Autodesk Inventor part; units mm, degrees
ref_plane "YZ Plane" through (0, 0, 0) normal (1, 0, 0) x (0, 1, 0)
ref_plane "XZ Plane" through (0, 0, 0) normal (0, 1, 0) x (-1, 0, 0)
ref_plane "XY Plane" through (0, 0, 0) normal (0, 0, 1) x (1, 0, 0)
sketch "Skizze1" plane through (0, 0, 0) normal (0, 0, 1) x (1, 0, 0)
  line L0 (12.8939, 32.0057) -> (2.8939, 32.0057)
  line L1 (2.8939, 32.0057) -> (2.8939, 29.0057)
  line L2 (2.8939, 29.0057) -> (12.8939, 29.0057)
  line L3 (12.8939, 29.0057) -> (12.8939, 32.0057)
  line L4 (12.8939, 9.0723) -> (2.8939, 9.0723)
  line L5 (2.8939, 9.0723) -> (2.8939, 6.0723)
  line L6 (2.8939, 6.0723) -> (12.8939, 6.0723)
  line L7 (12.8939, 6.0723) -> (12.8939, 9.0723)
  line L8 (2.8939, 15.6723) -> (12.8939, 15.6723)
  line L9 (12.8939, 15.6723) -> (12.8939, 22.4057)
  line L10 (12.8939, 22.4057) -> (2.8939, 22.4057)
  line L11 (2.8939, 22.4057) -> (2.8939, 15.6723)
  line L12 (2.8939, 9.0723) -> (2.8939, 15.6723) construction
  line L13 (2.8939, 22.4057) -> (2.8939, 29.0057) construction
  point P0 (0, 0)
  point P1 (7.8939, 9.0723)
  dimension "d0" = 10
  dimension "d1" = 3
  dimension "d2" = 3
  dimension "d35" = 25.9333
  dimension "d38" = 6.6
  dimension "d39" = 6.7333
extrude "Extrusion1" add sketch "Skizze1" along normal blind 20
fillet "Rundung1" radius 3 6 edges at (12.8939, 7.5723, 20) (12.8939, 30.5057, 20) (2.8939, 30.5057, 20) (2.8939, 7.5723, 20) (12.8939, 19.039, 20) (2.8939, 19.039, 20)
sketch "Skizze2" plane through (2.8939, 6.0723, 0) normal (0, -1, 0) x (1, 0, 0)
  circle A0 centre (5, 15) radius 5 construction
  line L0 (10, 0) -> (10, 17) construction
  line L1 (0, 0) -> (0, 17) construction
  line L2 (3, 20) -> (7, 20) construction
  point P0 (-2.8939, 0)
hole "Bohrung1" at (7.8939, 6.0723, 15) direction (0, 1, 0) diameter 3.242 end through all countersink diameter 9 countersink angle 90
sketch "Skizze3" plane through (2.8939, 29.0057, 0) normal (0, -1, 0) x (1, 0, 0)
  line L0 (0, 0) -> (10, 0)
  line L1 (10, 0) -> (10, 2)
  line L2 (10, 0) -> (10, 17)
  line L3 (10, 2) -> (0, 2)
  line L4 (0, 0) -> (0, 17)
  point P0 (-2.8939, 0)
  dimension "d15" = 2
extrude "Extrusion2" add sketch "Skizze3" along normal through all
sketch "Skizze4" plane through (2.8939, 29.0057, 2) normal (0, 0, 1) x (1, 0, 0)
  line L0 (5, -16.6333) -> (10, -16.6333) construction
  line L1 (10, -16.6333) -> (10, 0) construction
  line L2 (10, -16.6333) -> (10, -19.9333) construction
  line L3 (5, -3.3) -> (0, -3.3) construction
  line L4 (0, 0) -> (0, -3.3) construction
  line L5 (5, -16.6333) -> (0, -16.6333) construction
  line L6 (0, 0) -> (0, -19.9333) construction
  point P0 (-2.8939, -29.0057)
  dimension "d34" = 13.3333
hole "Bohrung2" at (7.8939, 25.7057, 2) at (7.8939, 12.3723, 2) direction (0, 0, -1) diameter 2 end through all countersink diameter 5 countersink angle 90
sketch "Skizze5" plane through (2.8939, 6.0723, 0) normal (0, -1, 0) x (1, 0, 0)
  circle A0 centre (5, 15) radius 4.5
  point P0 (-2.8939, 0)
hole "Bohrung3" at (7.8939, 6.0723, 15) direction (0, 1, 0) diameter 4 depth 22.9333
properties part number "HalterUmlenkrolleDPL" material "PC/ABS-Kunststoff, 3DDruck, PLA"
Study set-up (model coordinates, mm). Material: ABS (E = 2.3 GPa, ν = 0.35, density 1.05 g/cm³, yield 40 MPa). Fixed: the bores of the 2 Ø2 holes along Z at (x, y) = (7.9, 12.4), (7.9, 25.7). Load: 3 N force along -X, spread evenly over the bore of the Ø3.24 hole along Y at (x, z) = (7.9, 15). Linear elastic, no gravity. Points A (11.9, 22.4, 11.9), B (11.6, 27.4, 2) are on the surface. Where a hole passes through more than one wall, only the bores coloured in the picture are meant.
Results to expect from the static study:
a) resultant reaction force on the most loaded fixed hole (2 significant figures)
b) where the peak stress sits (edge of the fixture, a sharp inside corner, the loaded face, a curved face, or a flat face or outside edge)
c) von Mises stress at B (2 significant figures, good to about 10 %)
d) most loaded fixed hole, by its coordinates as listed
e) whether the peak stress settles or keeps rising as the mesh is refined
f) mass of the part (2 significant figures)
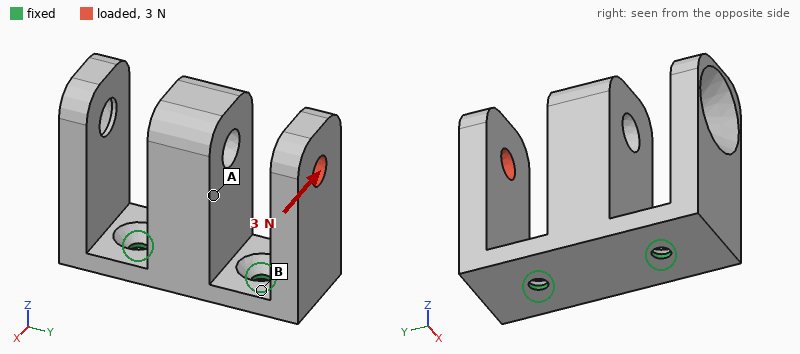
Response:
3.4 N
edge of the fixture
2.2 MPa
(7.9, 25.7)
keeps rising
2.7 g
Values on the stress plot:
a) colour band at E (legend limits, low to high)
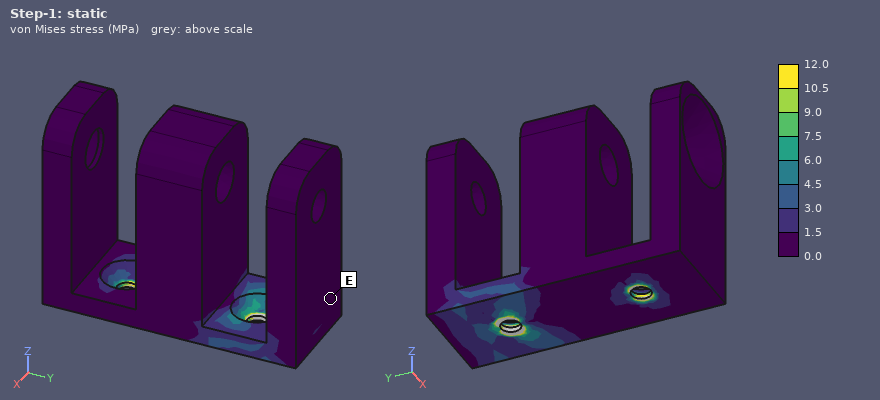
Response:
0.0 to 1.5 MPa
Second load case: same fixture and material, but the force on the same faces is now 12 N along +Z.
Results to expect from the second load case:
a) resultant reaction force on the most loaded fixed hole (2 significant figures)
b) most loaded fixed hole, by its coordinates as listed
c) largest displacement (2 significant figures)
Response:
18 N
(7.9, 25.7)
0.35 mm
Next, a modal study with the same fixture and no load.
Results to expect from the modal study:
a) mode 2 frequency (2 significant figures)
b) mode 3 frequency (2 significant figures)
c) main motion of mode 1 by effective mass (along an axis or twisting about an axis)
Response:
840 Hz
960 Hz
along X
